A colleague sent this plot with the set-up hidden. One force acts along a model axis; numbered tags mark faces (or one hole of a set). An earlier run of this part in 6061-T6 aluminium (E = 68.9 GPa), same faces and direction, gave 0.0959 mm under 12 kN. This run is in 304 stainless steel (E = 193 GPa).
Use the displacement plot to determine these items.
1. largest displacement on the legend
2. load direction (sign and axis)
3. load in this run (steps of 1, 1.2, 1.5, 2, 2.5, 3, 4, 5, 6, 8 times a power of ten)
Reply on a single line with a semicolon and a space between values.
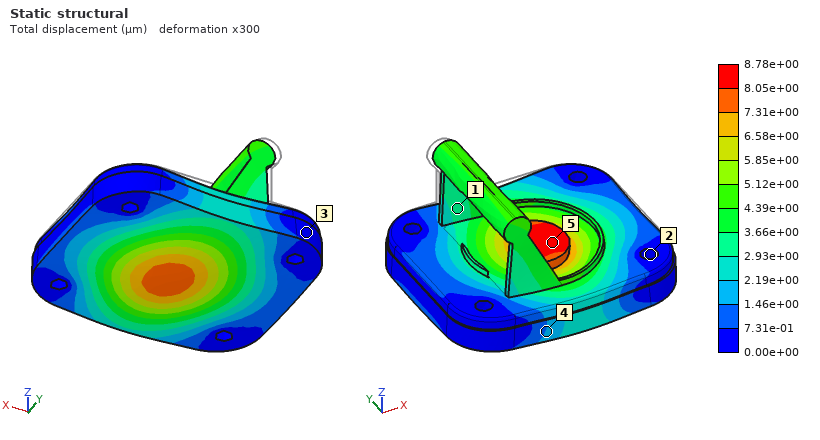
8.78e+00 µm; -Z; 3 kN
